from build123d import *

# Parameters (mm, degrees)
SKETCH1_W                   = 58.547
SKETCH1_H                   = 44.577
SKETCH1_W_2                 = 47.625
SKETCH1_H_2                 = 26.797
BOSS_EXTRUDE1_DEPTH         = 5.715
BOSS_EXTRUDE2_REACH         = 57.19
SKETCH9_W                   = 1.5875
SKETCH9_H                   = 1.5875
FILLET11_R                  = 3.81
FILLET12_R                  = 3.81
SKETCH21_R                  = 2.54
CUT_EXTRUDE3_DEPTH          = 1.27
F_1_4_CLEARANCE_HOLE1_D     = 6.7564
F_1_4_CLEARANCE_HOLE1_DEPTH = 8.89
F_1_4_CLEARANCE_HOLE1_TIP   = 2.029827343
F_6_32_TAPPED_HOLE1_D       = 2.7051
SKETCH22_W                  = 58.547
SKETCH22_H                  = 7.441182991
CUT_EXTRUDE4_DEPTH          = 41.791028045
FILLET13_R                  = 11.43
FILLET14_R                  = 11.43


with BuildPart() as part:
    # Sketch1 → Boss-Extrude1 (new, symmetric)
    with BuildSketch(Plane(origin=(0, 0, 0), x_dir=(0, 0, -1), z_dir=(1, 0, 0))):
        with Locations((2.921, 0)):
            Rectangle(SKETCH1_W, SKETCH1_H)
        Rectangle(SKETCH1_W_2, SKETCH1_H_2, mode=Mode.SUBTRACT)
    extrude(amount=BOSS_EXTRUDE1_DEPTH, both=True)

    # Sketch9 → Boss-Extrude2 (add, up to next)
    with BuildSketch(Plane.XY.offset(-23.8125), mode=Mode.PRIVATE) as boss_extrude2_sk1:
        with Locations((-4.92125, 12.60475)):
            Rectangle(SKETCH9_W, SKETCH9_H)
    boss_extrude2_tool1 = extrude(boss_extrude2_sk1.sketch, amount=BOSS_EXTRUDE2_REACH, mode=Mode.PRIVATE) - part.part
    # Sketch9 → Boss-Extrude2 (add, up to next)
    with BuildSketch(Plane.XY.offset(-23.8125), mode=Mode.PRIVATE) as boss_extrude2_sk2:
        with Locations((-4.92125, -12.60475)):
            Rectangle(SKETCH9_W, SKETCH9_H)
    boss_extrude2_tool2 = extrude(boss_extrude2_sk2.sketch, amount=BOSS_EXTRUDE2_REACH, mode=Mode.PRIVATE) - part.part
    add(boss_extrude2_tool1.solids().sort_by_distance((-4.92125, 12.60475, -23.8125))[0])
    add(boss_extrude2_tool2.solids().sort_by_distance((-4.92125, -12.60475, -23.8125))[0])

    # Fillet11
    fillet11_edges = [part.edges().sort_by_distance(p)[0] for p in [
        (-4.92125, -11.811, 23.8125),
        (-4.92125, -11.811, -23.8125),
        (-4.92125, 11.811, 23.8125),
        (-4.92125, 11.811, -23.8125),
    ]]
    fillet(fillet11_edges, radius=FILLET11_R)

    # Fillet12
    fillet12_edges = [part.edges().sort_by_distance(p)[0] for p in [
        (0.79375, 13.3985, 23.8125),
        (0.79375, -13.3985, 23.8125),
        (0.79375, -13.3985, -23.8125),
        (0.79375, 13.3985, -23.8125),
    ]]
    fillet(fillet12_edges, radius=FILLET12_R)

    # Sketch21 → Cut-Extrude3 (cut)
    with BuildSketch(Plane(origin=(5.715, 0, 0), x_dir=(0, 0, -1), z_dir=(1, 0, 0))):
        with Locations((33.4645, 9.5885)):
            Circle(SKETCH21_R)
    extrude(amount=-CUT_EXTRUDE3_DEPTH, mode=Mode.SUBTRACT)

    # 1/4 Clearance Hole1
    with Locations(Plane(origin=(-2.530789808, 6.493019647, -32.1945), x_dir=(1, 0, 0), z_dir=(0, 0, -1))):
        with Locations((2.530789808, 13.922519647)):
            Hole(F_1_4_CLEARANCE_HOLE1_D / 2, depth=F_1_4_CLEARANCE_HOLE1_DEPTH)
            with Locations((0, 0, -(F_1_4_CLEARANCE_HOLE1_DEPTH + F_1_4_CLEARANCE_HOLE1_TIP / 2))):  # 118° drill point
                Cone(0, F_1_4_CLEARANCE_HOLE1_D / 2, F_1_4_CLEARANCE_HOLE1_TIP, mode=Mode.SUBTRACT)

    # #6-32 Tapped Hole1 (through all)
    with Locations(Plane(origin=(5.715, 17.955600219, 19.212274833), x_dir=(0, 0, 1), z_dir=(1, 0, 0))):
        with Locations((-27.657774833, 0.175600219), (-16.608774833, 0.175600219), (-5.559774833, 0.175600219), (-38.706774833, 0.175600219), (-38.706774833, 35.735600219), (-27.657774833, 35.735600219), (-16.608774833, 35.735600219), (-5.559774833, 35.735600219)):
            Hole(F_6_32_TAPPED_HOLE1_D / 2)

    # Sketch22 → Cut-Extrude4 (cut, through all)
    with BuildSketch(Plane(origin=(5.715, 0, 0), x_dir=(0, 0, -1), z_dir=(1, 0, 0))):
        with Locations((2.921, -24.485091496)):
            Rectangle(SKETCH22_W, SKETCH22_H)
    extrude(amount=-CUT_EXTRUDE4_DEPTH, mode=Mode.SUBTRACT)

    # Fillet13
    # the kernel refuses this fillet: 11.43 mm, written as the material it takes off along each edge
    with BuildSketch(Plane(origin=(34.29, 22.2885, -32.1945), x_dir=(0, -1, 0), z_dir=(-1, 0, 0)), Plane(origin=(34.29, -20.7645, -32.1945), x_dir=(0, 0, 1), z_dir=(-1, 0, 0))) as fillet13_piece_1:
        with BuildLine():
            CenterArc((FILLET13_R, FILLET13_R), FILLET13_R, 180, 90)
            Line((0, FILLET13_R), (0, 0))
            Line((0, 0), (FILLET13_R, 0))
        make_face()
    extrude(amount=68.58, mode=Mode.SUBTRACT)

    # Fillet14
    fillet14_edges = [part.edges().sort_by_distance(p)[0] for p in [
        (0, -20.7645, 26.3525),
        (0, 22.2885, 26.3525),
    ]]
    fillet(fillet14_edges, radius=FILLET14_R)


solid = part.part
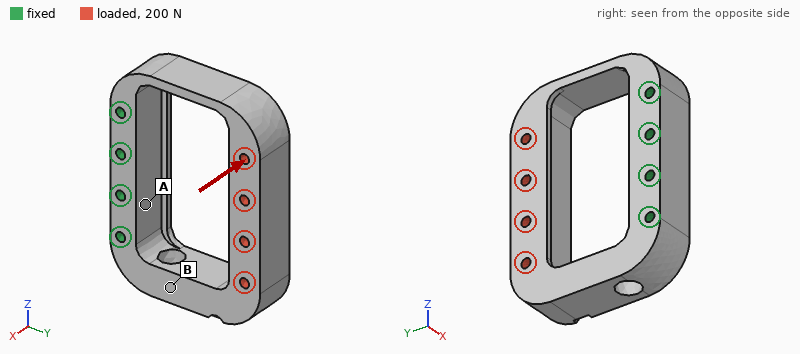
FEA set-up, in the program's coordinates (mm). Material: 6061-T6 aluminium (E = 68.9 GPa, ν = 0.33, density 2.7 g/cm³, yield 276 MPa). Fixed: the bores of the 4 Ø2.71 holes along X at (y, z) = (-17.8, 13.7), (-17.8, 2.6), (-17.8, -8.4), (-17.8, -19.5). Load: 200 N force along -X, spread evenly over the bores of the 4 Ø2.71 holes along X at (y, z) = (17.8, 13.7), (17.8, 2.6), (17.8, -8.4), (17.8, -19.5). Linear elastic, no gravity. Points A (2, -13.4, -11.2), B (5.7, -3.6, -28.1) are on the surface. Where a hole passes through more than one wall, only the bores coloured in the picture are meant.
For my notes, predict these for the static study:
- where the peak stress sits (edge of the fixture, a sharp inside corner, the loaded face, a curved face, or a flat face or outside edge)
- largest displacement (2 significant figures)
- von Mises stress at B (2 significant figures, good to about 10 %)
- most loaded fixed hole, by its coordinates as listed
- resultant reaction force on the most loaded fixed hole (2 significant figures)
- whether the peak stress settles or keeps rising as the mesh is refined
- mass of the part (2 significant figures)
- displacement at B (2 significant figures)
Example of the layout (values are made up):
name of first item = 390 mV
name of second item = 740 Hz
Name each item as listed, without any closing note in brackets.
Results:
where the peak stress sits = edge of the fixture
largest displacement = 99 µm
von Mises stress at B = 15 MPa
most loaded fixed hole, by its coordinates as listed = (-17.8, -19.5)
resultant reaction force on the most loaded fixed hole = 98 N
whether the peak stress settles or keeps rising as the mesh is refined = keeps rising
mass of the part = 34 g
displacement at B = 20 µm
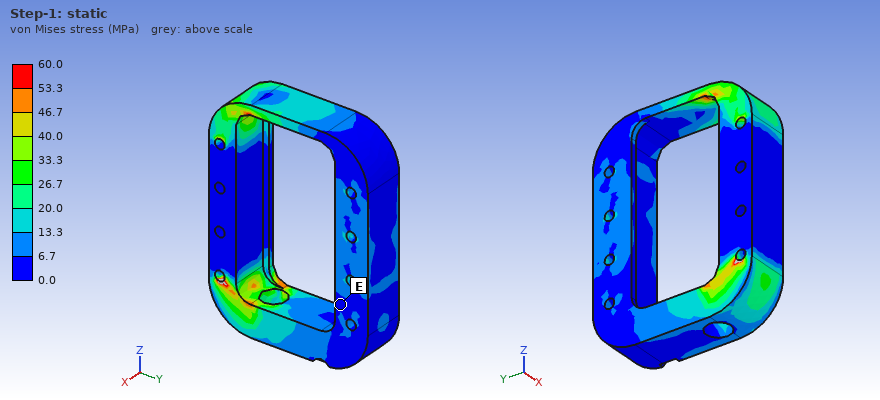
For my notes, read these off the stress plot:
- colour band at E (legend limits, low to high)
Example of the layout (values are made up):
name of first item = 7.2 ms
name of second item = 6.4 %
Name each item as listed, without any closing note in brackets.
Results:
colour band at E = 0.0 to 6.7 MPa
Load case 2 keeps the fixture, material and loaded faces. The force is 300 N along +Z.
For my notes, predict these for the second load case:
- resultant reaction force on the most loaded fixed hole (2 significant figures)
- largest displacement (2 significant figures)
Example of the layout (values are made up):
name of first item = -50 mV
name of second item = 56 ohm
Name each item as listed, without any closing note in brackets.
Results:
resultant reaction force on the most loaded fixed hole = 320 N
largest displacement = 78 µm
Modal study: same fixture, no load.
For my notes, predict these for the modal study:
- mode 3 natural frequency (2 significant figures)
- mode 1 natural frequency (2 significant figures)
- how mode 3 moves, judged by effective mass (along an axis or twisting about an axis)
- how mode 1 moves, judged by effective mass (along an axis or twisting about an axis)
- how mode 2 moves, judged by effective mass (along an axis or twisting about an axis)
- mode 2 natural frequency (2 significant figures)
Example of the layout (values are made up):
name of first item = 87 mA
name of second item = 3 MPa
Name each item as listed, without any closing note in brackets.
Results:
mode 3 natural frequency = 4800 Hz
mode 1 natural frequency = 2000 Hz
how mode 3 moves, judged by effective mass = twisting about Y
how mode 1 moves, judged by effective mass = along X
how mode 2 moves, judged by effective mass = along Z
mode 2 natural frequency = 2400 Hz
